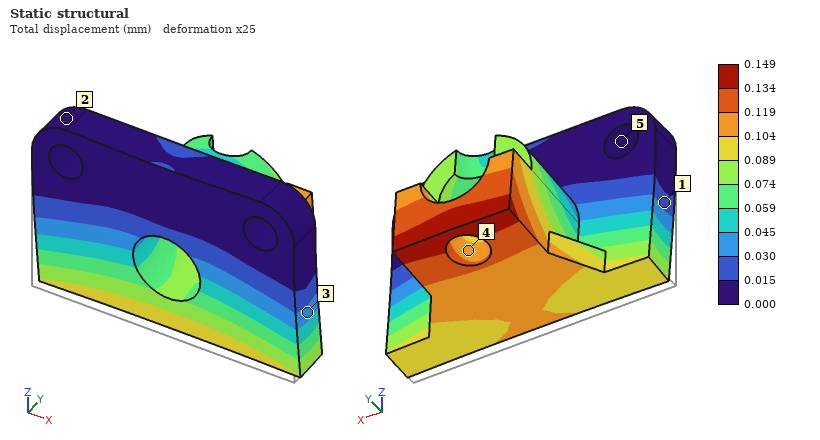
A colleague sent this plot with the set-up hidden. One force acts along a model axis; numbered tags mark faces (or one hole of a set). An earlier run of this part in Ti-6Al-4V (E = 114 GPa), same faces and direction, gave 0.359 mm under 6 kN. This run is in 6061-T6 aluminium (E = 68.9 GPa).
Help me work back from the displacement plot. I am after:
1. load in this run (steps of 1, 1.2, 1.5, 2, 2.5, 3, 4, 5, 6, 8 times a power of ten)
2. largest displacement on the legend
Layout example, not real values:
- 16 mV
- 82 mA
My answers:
- 1.5 kN
- 0.149 mm
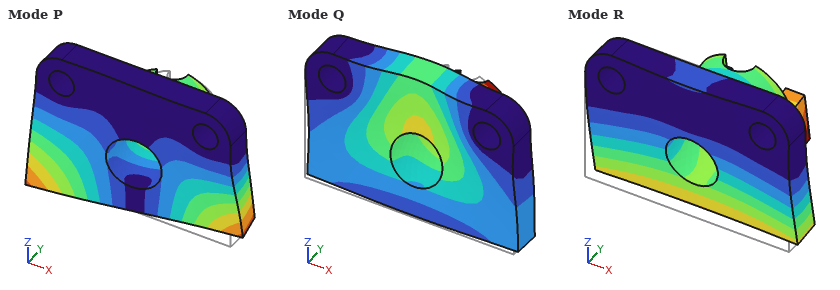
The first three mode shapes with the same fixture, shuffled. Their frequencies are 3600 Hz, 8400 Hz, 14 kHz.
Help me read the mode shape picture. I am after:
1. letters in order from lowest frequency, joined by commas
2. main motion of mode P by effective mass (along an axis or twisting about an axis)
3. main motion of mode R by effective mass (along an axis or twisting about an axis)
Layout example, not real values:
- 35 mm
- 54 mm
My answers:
- R, P, Q
- along X
- along Y
